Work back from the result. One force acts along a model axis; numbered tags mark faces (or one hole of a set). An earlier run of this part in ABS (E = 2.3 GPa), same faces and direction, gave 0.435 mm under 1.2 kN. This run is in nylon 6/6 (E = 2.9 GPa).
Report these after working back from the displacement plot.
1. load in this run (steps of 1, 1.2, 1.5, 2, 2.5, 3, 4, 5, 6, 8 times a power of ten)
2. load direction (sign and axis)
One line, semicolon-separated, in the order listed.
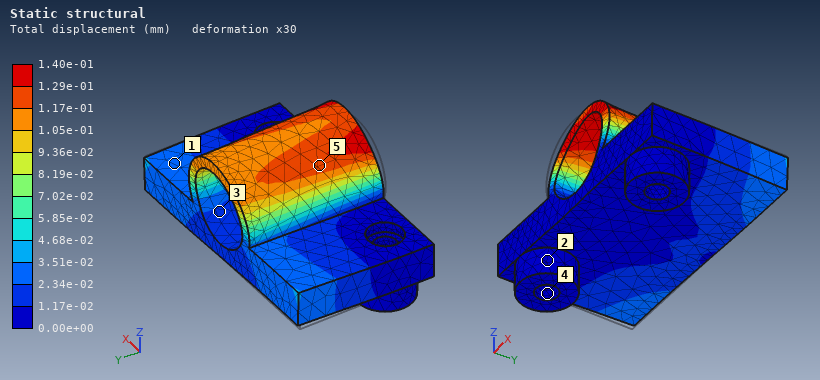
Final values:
500 N; +X
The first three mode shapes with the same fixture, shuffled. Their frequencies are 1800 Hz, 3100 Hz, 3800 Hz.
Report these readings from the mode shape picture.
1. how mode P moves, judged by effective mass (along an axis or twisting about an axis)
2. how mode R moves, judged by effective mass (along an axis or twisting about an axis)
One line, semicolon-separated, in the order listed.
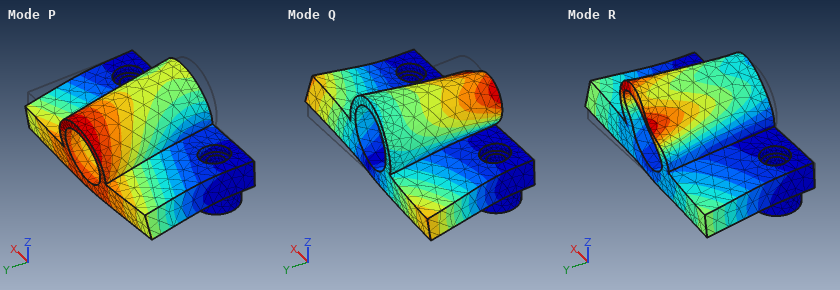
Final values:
along Z; along X
